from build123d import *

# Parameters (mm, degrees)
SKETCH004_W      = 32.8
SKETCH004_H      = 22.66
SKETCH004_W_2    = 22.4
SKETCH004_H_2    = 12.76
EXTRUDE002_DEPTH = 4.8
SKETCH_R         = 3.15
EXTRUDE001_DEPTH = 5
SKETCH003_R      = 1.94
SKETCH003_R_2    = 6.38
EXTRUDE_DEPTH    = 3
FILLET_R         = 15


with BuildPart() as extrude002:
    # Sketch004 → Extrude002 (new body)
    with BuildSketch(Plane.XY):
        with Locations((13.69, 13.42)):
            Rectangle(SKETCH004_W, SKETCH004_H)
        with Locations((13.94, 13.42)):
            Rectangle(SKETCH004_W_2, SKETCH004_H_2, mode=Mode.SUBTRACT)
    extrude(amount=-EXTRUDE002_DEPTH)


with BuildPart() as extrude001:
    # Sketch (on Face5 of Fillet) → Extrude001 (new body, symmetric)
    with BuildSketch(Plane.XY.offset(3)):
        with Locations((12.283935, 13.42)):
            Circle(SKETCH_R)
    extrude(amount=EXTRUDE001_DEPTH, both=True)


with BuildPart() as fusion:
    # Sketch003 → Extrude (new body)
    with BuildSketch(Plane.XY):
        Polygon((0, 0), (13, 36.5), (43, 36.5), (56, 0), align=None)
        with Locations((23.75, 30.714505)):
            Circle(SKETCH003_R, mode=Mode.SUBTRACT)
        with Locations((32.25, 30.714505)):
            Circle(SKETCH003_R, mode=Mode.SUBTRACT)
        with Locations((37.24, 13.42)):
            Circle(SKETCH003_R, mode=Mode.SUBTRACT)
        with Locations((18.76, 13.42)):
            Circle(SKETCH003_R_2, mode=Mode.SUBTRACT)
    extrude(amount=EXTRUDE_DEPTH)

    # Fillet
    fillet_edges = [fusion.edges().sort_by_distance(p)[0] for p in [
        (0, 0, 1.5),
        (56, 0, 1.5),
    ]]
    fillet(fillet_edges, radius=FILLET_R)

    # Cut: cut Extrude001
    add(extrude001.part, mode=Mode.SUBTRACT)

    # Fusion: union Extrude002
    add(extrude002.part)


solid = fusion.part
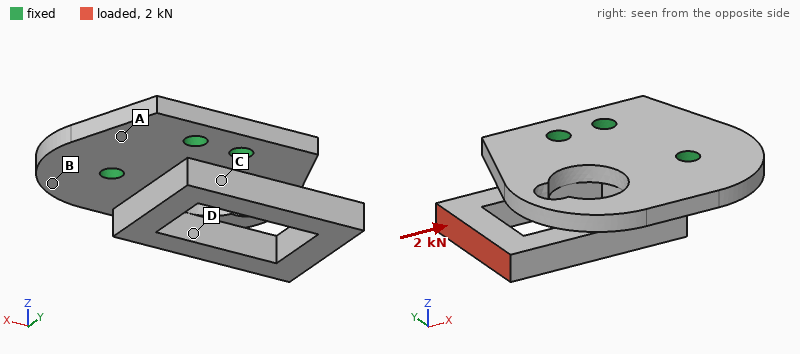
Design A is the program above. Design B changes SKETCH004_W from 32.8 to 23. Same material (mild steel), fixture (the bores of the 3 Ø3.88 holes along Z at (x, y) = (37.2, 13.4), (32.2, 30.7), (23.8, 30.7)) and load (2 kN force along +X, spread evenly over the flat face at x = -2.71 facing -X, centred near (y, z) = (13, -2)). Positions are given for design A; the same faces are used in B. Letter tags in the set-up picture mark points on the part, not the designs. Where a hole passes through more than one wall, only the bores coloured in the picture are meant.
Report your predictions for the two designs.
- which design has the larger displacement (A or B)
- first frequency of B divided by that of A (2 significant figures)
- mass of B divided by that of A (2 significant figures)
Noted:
B
1.1
0.81
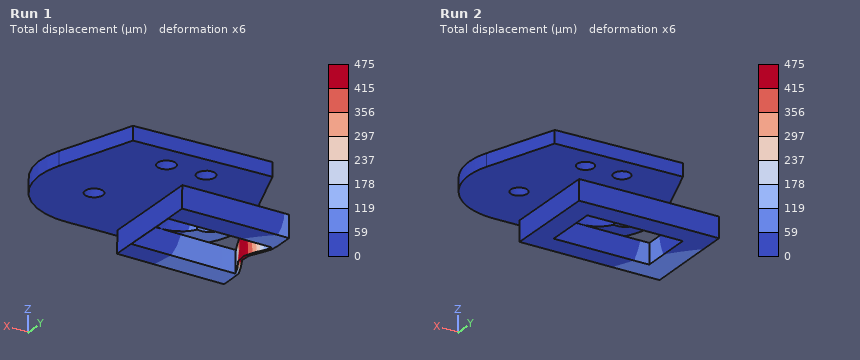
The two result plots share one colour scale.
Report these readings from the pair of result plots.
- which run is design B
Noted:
Run 1
